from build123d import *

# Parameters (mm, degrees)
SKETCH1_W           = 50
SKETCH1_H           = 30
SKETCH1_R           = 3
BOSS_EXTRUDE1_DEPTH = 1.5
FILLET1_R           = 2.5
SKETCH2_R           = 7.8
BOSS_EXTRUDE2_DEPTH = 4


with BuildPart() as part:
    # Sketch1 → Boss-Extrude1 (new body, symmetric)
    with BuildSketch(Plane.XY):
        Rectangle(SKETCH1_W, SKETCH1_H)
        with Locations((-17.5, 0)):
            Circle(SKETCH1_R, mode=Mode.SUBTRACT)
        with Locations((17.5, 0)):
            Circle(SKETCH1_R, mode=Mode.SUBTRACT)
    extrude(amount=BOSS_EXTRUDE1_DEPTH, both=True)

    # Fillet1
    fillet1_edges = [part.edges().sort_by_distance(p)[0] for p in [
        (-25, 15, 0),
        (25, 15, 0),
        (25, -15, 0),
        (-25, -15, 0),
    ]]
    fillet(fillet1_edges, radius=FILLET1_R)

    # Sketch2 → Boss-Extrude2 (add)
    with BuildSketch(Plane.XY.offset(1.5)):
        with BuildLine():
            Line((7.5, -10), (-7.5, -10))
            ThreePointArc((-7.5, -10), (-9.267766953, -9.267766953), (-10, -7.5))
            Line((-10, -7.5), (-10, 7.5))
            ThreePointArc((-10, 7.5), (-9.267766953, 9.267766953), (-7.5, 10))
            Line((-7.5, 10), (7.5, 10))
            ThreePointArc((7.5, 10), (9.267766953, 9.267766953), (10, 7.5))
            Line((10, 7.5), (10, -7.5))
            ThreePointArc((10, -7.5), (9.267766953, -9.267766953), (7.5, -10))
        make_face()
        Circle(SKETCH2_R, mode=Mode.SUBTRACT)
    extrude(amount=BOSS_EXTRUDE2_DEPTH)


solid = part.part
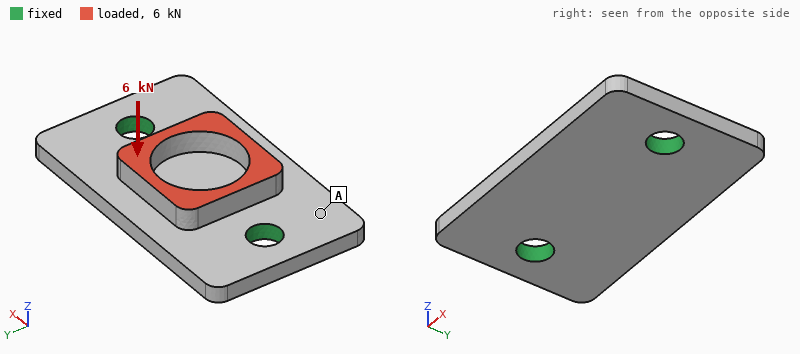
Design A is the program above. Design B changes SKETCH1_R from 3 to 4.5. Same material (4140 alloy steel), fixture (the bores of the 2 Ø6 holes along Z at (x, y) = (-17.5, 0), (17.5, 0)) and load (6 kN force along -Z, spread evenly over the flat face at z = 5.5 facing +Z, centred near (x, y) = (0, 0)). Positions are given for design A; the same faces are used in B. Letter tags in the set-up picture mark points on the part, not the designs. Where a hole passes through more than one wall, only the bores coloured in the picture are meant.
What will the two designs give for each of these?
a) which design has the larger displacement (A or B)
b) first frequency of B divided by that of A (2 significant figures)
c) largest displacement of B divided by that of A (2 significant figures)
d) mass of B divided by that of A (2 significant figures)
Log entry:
A
1.3
0.69
0.96
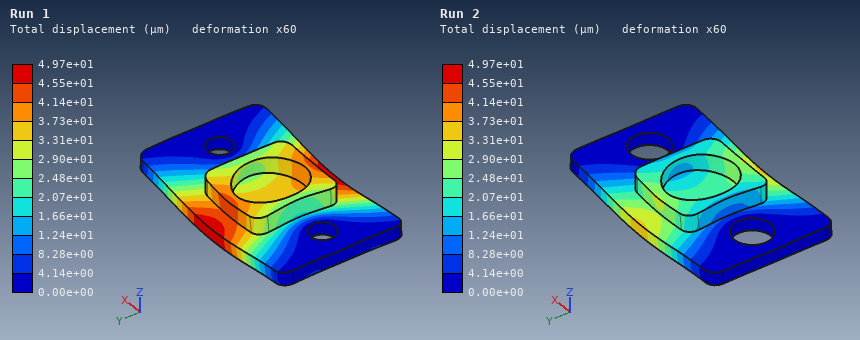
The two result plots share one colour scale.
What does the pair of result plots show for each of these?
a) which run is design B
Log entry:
Run 2
